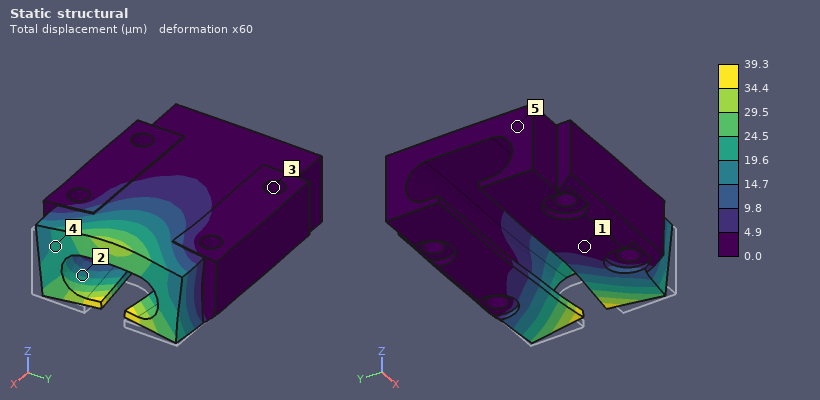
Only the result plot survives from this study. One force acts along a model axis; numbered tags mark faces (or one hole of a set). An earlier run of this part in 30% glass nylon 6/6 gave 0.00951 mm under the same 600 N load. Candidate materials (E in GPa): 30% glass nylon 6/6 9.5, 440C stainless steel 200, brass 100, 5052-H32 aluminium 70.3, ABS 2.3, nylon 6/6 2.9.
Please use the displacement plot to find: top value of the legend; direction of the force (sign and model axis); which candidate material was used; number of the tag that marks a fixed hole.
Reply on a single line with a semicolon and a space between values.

39.3 µm; -X; ABS; 3
